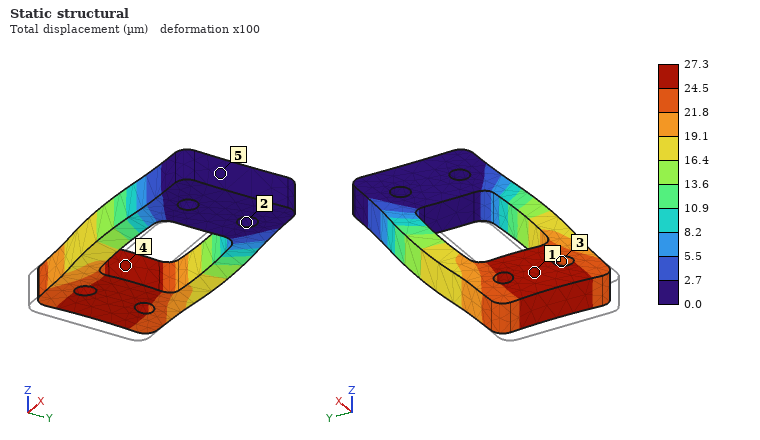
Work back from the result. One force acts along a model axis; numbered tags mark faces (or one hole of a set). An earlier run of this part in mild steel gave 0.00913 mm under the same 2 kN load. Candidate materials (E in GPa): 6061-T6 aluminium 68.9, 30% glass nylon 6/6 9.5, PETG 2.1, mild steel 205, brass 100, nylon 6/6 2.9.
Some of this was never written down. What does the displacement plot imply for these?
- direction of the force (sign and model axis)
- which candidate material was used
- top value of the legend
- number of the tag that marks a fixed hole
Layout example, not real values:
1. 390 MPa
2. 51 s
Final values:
1. +X
2. 6061-T6 aluminium
3. 27.3 µm
4. 2
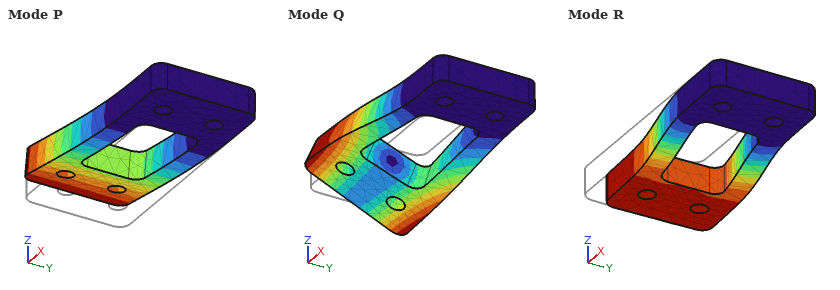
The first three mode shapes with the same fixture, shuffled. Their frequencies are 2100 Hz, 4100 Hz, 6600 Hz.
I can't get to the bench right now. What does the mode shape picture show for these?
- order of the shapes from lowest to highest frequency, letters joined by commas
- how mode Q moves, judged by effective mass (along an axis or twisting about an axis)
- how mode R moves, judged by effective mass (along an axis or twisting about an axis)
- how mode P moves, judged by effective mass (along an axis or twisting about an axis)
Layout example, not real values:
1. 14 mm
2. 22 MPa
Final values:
1. P, R, Q
2. twisting about X
3. along Y
4. along Z
